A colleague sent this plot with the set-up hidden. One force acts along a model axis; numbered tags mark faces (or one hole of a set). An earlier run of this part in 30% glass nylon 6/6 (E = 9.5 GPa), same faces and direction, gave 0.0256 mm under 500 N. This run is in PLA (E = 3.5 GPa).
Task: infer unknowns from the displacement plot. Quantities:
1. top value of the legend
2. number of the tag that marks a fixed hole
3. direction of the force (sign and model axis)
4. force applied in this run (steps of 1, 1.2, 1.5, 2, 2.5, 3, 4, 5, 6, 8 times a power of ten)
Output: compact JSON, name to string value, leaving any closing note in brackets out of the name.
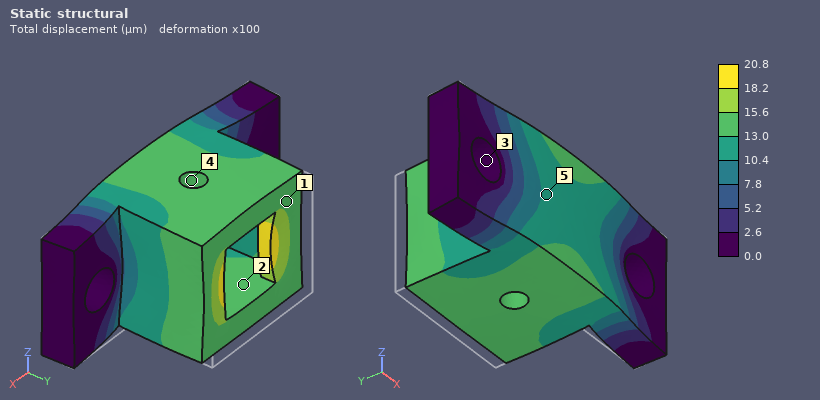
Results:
{"top value of the legend": "20.8 µm", "number of the tag that marks a fixed hole": "3", "direction of the force": "-Y", "force applied in this run": "150 N"}
